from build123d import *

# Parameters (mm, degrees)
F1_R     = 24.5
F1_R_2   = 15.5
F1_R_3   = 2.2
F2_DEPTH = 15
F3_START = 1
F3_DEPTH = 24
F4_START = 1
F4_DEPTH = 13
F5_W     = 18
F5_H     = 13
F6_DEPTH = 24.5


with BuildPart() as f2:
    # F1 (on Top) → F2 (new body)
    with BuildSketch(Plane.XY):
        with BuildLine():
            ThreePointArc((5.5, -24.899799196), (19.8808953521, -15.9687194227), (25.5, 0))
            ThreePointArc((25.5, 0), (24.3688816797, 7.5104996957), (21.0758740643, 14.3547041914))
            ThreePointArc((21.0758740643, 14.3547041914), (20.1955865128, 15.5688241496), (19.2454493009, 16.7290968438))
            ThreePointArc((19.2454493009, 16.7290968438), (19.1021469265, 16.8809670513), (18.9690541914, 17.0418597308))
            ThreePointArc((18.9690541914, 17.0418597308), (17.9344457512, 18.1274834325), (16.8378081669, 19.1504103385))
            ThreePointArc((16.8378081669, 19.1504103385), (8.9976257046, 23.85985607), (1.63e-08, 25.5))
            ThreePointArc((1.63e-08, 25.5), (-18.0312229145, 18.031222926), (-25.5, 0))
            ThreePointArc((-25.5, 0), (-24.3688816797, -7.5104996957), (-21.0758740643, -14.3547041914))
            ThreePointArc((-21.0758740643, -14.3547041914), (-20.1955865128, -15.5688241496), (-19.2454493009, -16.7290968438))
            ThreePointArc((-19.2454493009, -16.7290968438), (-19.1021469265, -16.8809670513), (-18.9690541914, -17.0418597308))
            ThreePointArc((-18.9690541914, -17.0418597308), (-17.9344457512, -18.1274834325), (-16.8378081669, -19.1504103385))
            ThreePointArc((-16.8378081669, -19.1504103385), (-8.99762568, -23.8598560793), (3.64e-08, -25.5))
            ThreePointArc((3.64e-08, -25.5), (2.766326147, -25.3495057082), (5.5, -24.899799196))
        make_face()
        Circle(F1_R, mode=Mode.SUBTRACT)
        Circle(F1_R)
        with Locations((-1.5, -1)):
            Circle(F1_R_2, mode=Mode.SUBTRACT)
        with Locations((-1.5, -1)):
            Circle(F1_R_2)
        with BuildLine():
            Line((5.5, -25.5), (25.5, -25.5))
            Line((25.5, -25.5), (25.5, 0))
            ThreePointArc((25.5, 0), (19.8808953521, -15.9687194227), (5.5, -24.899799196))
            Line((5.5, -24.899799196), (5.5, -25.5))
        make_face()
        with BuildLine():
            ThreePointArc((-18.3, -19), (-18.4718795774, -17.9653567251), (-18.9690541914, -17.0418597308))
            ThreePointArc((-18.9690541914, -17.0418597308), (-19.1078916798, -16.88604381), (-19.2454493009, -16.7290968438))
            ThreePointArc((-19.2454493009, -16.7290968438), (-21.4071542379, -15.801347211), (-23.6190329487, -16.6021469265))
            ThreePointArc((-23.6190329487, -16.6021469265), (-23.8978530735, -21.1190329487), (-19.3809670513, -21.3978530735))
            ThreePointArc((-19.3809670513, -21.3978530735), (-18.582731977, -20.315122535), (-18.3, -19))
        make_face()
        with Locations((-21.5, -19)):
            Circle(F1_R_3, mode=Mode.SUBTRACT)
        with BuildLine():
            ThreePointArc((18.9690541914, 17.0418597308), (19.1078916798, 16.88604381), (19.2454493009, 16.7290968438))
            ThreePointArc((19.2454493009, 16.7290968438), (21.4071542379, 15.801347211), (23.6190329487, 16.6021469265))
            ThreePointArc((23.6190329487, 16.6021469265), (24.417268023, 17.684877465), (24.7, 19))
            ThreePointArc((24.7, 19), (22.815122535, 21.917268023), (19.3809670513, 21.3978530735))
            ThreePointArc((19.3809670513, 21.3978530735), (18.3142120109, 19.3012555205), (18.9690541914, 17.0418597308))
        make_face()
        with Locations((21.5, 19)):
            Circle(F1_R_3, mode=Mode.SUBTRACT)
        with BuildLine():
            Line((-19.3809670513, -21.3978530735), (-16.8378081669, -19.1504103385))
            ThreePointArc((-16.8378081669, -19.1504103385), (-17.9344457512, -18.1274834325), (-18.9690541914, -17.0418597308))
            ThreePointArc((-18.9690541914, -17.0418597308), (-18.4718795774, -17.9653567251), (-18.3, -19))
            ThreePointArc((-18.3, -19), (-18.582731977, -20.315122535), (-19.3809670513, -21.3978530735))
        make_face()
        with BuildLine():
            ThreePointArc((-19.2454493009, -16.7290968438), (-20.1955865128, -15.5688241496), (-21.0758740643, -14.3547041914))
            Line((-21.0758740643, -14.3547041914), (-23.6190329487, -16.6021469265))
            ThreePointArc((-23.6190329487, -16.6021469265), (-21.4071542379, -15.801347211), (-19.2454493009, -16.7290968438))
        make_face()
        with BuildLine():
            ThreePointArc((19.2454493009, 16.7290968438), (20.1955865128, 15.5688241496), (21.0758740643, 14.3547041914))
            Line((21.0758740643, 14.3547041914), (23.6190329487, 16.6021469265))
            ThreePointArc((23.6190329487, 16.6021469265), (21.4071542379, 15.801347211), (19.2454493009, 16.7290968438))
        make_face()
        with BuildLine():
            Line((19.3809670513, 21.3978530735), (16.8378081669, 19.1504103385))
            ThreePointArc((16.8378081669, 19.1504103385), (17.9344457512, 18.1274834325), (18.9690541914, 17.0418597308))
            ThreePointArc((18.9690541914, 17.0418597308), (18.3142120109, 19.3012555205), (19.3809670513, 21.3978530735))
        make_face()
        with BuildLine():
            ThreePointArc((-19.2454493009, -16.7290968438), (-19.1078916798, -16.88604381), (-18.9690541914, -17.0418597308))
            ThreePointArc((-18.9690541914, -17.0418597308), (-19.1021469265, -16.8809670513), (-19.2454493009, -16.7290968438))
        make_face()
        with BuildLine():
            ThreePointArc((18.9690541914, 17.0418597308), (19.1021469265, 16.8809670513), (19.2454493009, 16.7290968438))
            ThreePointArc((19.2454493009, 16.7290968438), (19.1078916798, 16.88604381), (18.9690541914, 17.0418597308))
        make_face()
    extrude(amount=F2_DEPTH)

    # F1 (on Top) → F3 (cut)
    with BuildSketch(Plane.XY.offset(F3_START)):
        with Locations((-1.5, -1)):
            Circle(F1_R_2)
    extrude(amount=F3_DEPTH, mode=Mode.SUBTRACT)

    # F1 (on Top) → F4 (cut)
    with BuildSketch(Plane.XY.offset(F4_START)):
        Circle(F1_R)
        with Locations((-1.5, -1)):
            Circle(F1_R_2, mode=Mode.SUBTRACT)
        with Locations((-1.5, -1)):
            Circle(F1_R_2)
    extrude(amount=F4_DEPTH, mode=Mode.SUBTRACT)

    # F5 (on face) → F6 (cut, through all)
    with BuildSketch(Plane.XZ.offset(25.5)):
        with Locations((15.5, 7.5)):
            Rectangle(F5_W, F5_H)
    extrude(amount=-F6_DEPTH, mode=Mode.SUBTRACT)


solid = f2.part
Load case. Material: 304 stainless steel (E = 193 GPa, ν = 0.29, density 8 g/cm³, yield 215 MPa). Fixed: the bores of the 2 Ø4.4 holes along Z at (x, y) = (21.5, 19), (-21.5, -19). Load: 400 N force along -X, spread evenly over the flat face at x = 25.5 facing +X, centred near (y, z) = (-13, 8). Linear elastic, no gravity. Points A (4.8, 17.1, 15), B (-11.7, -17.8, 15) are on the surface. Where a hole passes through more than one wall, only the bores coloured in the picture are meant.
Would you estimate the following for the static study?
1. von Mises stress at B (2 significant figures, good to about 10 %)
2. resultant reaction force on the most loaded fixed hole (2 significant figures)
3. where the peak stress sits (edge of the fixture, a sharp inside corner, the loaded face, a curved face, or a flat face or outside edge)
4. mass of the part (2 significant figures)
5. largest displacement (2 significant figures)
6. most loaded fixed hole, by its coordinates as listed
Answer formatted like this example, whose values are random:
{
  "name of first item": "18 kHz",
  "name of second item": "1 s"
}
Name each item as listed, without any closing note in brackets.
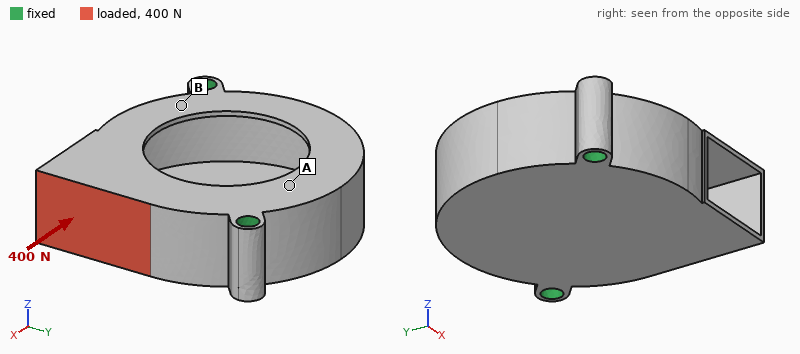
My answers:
{
  "von Mises stress at B": "22 MPa",
  "resultant reaction force on the most loaded fixed hole": "290 N",
  "where the peak stress sits": "a flat face or outside edge",
  "mass of the part": "50 g",
  "largest displacement": "21 µm",
  "most loaded fixed hole, by its coordinates as listed": "(-21.5, -19)"
}
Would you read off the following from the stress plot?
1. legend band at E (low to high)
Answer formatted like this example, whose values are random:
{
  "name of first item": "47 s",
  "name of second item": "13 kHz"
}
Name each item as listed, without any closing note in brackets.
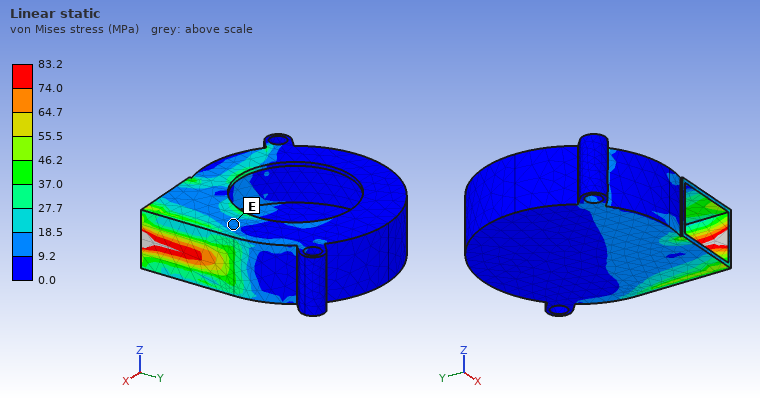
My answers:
{
  "legend band at E": "9.2 to 18.5 MPa"
}
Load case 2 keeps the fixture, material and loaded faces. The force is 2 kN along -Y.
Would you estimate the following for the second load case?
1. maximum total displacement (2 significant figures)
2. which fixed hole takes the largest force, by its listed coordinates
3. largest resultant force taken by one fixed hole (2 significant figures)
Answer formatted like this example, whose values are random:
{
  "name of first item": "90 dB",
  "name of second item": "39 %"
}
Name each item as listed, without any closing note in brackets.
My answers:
{
  "maximum total displacement": "22 µm",
  "which fixed hole takes the largest force, by its listed coordinates": "(21.5, 19)",
  "largest resultant force taken by one fixed hole": "1.9 kN"
}
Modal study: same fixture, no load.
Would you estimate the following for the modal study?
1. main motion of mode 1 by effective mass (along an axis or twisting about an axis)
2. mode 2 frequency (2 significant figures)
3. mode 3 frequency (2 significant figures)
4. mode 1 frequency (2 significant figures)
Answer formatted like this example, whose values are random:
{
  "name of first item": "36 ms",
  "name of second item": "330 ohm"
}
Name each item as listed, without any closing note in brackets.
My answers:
{
  "main motion of mode 1 by effective mass": "along Z",
  "mode 2 frequency": "5500 Hz",
  "mode 3 frequency": "5800 Hz",
  "mode 1 frequency": "3300 Hz"
}
